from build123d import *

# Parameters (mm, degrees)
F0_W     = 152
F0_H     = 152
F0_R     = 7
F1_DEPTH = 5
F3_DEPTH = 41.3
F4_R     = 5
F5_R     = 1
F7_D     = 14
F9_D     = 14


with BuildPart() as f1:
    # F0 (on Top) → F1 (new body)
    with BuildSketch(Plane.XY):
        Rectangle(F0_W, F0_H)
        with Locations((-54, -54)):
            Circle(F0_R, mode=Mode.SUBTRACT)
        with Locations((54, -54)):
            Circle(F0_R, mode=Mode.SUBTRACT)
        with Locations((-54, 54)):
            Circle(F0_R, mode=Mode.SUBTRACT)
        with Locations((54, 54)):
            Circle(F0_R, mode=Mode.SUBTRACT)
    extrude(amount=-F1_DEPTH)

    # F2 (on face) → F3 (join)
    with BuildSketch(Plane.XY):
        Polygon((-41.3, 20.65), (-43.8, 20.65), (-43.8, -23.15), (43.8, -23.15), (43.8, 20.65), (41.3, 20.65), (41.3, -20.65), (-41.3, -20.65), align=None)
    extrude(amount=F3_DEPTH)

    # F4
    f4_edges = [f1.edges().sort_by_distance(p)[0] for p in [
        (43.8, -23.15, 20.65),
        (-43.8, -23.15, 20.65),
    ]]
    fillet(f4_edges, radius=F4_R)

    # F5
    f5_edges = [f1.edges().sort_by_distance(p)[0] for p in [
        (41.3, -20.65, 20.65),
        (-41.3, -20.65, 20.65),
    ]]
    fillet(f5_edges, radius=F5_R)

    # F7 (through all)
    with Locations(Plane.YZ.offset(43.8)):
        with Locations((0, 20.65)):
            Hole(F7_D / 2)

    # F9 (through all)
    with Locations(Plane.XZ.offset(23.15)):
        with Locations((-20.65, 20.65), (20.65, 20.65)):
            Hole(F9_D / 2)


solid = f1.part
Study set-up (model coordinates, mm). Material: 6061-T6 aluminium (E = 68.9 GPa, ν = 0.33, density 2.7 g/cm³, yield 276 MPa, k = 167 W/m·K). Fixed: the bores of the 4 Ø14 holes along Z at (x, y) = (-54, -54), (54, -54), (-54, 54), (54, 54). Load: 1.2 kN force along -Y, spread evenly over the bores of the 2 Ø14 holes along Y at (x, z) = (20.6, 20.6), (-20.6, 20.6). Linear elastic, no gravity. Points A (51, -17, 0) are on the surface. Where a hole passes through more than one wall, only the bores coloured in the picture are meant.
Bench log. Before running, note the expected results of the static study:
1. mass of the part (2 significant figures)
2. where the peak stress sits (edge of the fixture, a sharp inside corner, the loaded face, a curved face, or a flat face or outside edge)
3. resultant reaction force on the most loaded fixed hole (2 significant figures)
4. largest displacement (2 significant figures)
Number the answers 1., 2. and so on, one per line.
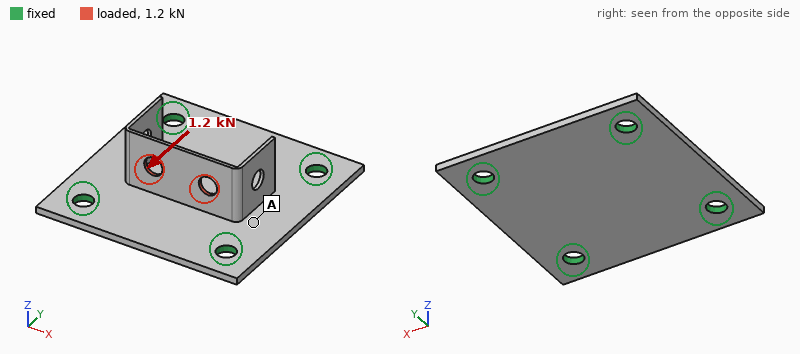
1. 350 g
2. the loaded face
3. 370 N
4. 0.54 mm
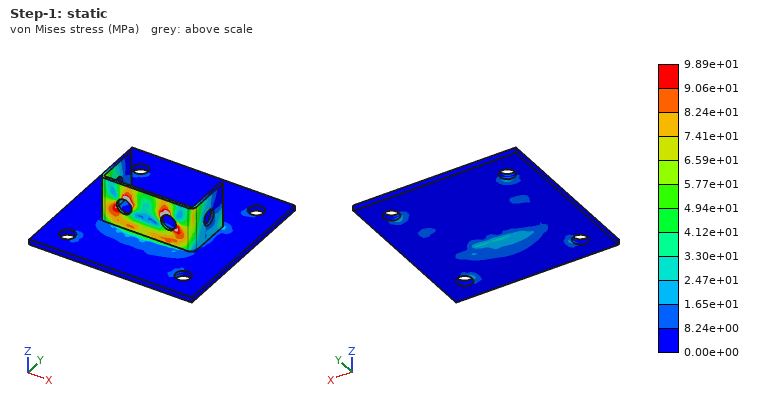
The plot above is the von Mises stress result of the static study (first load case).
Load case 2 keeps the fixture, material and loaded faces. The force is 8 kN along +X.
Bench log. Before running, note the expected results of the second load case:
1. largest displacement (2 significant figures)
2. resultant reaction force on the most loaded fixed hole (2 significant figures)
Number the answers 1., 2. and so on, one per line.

1. 0.29 mm
2. 3.3 kN
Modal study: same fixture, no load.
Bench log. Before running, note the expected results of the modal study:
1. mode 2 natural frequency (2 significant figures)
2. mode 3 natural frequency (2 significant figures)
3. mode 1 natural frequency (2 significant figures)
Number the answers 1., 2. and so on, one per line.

1. 1900 Hz
2. 2000 Hz
3. 1700 Hz
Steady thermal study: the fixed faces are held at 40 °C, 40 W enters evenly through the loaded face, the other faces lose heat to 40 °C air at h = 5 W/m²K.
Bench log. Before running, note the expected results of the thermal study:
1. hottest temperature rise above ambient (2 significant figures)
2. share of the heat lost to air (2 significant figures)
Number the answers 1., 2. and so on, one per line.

1. 37 K
2. 5.7 %
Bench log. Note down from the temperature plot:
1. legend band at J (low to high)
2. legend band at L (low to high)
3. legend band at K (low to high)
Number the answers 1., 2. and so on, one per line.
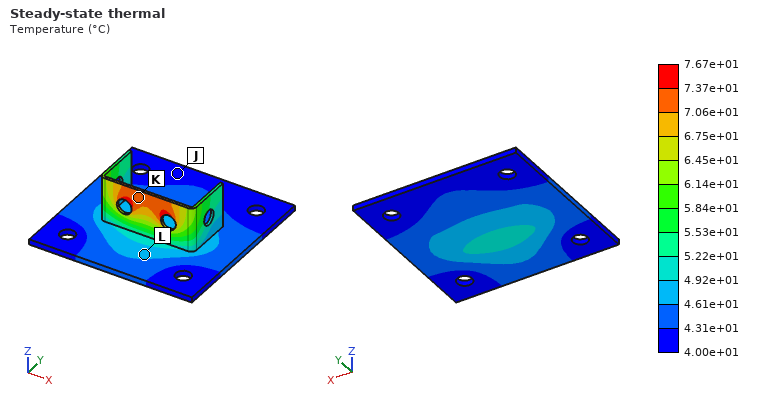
1. 4.00e+01 to 4.31e+01 °C
2. 4.61e+01 to 4.92e+01 °C
3. 7.06e+01 to 7.37e+01 °C
